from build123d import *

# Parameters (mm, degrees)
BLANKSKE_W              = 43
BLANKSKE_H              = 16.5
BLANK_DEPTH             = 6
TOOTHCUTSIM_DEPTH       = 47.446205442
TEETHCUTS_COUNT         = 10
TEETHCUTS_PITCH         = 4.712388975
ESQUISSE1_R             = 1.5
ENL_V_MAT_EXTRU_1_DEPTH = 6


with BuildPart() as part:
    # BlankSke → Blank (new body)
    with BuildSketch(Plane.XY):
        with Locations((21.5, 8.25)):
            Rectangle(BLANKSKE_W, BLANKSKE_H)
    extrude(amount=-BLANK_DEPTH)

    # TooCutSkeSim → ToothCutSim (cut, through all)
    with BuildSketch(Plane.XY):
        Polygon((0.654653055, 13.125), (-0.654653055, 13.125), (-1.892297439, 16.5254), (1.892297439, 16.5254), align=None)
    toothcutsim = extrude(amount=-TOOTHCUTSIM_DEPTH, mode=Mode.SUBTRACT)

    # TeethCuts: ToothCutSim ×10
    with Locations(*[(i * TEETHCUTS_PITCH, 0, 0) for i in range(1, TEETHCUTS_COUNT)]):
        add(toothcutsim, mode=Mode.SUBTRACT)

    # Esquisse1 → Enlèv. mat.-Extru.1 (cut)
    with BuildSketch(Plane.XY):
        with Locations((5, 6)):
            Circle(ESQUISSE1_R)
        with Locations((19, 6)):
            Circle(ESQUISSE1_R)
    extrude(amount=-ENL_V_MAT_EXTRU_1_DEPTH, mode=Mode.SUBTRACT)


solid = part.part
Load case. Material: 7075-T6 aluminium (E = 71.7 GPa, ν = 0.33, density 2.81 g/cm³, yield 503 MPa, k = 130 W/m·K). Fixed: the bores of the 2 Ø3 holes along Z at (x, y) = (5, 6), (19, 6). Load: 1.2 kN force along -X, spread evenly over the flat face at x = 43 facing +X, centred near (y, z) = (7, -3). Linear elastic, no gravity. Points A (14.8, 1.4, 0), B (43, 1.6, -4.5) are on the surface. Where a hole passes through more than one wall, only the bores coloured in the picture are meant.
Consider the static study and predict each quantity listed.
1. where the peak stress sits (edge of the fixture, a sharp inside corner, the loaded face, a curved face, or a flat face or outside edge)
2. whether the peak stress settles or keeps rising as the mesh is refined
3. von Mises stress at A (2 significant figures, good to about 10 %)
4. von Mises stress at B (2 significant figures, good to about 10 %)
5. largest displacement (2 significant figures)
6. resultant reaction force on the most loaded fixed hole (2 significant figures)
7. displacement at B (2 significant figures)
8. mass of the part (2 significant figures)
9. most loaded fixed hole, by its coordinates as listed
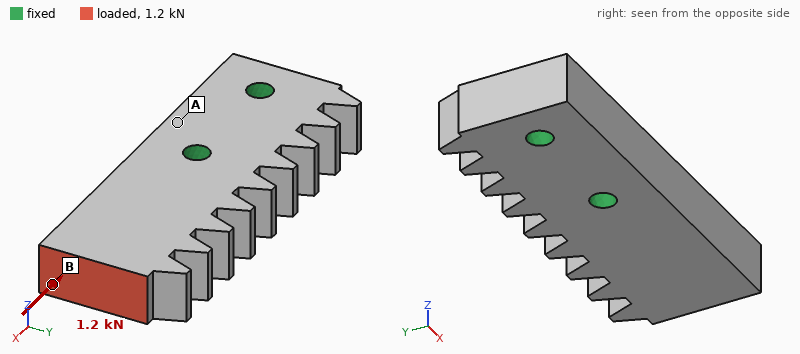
edge of the fixture
keeps rising
4.6 MPa
15 MPa
5.6 µm
1.0 kN
5.4 µm
10 g
(19, 6)
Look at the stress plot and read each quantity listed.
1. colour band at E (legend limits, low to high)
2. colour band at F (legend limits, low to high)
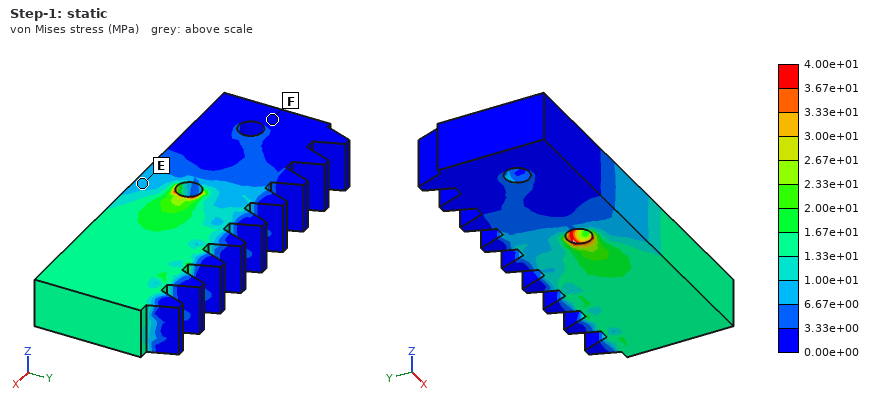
6.67e+00 to 1.00e+01 MPa
0.00e+00 to 3.33e+00 MPa
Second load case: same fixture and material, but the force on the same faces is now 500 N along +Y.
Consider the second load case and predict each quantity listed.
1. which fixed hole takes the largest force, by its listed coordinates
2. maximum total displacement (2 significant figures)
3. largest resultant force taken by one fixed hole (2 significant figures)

(19, 6)
54 µm
1.1 kN
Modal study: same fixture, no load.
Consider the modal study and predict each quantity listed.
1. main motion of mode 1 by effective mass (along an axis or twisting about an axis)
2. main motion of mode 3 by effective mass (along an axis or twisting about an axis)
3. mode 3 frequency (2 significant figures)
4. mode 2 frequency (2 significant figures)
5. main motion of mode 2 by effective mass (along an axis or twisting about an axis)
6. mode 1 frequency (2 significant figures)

along Z
twisting about X
19 kHz
11 kHz
along Y
7600 Hz
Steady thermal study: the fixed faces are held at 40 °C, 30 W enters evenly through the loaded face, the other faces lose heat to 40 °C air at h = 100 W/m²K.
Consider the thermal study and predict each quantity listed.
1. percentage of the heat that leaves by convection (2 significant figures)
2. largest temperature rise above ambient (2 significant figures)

12 %
65 K
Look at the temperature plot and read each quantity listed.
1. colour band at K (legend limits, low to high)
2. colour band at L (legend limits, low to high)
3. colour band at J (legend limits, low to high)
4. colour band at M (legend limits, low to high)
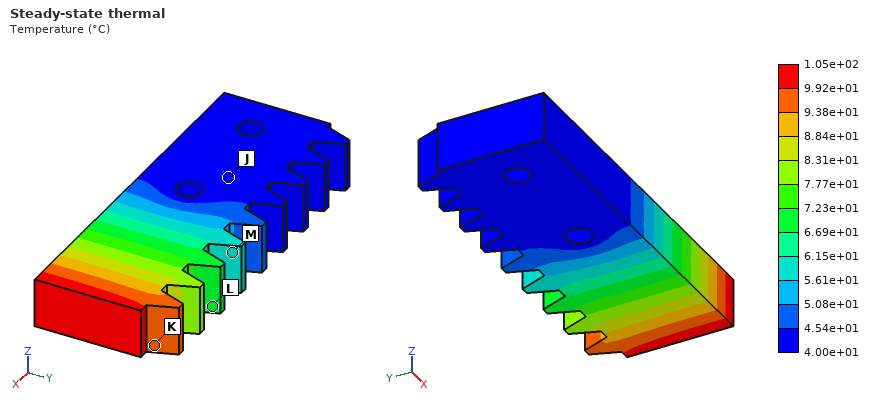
9.38e+01 to 9.92e+01 °C
6.69e+01 to 7.23e+01 °C
4.00e+01 to 4.54e+01 °C
5.61e+01 to 6.15e+01 °C
